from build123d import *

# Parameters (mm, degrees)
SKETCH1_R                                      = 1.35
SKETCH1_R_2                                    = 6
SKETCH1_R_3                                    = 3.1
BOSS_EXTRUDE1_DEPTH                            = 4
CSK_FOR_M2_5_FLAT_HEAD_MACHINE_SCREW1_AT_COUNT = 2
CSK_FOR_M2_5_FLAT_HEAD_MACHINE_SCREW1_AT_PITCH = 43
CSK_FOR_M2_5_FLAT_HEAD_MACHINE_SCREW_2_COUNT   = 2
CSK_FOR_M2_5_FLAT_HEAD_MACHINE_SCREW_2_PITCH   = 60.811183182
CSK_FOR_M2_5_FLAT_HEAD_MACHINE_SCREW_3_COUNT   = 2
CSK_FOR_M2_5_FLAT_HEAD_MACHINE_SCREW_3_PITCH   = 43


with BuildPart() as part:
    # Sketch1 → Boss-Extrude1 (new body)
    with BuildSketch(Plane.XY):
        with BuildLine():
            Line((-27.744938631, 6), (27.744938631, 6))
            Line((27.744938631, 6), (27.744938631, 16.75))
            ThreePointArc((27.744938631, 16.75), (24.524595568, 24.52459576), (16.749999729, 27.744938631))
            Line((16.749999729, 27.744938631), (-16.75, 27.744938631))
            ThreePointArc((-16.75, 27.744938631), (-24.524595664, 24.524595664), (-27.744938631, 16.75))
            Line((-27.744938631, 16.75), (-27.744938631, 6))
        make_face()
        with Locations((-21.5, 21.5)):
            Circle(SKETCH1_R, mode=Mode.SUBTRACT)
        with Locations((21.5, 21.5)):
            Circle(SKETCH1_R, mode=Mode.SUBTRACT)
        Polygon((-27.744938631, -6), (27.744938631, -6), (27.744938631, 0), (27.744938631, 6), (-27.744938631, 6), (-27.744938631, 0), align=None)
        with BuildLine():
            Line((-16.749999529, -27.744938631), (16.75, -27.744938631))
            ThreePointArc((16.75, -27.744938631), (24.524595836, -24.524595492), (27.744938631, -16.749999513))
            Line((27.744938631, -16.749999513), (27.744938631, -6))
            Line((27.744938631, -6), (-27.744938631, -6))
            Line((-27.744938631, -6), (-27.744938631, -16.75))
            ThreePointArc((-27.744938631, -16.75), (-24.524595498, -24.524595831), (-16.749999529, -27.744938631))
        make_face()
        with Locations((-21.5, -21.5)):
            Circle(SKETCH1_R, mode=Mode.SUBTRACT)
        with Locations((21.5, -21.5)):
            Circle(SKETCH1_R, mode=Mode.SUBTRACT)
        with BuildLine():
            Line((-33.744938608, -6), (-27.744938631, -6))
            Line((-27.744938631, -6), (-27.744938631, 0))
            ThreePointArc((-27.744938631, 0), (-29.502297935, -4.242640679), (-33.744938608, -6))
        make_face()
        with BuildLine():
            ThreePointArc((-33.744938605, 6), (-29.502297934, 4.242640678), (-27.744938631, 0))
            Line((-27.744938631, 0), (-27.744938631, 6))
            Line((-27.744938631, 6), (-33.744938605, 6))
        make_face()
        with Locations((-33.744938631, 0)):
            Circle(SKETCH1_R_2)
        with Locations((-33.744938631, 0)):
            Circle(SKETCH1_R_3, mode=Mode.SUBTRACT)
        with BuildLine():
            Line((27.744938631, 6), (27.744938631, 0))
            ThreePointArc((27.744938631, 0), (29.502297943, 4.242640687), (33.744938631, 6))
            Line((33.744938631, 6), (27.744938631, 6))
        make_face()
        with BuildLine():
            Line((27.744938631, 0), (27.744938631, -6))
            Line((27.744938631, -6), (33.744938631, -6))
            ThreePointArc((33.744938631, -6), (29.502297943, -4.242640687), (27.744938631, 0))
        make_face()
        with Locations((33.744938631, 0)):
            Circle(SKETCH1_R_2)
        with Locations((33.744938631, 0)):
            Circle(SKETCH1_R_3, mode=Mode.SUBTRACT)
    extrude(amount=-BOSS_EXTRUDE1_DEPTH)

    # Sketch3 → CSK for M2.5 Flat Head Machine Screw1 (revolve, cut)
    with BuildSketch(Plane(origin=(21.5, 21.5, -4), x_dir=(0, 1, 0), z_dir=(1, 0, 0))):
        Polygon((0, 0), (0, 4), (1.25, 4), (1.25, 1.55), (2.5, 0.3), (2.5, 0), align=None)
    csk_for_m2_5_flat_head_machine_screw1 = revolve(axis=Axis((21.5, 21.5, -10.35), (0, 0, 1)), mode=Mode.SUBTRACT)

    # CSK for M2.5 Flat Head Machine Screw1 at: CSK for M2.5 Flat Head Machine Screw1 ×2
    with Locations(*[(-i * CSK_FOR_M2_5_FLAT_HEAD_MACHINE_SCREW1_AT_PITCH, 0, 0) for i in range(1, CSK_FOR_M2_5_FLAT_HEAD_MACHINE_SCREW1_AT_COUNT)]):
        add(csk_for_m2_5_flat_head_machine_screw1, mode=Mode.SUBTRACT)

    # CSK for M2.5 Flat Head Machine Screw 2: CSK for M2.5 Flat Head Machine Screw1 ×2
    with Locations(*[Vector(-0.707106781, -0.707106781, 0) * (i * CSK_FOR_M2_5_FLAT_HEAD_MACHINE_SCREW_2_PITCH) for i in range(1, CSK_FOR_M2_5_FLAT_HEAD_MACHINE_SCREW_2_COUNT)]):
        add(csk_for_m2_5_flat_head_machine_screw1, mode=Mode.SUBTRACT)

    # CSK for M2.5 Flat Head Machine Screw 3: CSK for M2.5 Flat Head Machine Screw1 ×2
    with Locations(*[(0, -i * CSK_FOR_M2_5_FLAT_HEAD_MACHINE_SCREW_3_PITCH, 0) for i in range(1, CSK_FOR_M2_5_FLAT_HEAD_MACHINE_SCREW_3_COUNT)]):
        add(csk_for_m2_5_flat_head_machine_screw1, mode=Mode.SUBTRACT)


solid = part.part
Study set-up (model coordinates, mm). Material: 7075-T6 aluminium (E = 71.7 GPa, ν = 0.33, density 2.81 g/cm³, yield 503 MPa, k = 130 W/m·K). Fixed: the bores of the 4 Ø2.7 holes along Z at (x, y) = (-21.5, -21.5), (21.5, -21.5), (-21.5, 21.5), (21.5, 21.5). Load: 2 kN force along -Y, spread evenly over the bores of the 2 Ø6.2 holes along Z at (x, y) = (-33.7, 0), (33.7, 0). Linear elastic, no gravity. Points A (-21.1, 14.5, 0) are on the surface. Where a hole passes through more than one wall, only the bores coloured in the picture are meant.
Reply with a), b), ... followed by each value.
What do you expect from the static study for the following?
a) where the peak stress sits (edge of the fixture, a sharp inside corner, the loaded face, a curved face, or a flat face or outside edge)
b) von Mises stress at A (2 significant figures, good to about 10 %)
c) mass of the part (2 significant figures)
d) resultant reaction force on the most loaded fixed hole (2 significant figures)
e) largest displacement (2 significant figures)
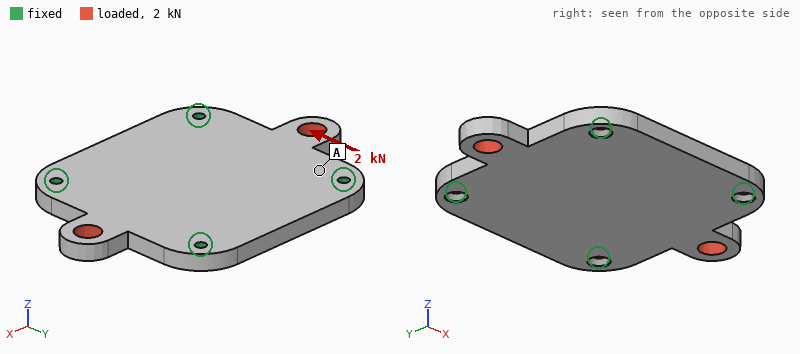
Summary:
a) the loaded face
b) 16 MPa
c) 35 g
d) 520 N
e) 38 µm
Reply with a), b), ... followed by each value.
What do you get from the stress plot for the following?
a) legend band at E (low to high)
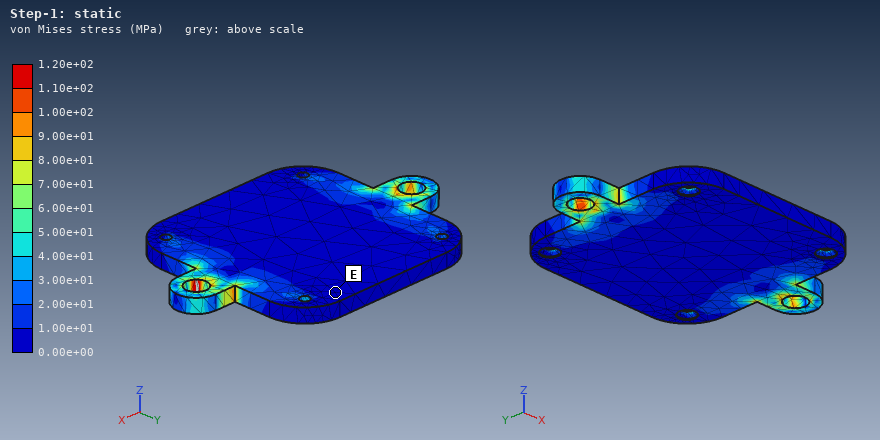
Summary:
a) 0.00e+00 to 1.00e+01 MPa
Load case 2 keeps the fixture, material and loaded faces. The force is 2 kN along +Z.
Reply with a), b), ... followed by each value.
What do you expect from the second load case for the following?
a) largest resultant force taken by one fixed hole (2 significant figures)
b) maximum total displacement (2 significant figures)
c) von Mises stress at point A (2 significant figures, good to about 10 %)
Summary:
a) 690 N
b) 0.51 mm
c) 120 MPa
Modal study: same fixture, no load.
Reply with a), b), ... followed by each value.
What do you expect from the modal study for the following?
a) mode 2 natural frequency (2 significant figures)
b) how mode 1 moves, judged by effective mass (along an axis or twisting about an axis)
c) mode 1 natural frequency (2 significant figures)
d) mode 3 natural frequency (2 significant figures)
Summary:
a) 7000 Hz
b) along Z
c) 6300 Hz
d) 7100 Hz
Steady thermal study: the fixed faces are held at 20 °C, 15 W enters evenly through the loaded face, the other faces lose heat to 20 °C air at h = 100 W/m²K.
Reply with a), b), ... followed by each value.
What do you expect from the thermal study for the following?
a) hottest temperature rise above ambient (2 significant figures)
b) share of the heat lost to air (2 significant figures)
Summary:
a) 23 K
b) 22 %
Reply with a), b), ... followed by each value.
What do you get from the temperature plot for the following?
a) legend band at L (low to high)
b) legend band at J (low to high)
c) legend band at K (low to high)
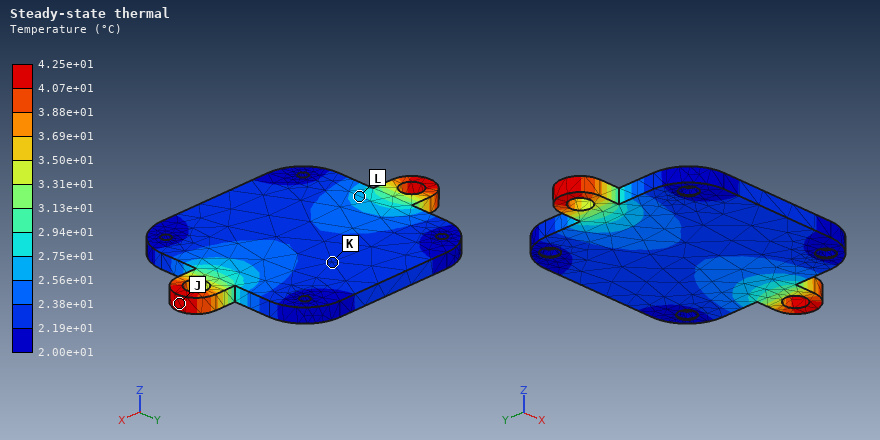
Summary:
a) 2.56e+01 to 2.75e+01 °C
b) 4.07e+01 to 4.25e+01 °C
c) 2.19e+01 to 2.38e+01 °C
